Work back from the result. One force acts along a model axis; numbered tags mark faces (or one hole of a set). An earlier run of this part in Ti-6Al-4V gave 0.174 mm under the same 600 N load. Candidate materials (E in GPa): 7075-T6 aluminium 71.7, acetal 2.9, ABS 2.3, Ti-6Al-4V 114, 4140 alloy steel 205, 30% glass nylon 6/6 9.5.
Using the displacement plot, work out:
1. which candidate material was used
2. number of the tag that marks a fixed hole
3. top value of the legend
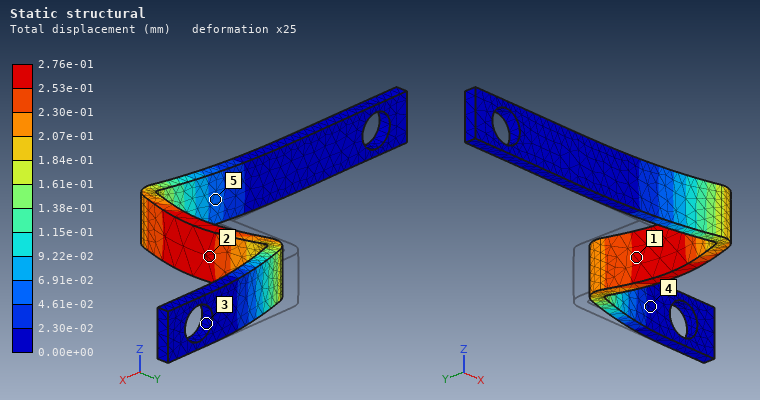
7075-T6 aluminium
3
2.76e-01 mm
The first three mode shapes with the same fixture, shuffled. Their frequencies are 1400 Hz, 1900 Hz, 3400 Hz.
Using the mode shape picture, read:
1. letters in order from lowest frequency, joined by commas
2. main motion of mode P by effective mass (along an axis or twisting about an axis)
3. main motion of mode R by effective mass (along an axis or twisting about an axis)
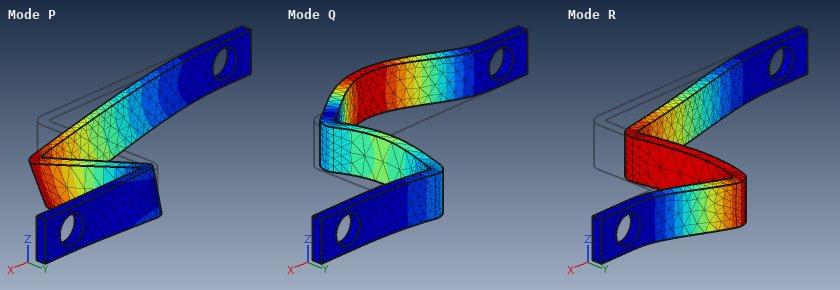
R, P, Q
along Z
along Y
